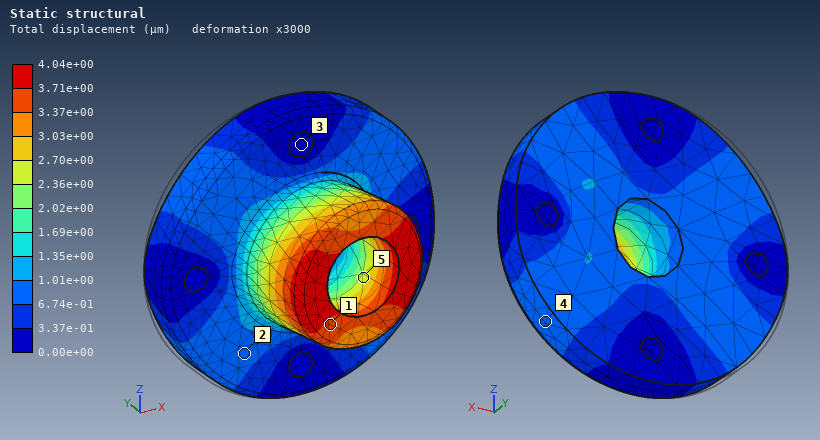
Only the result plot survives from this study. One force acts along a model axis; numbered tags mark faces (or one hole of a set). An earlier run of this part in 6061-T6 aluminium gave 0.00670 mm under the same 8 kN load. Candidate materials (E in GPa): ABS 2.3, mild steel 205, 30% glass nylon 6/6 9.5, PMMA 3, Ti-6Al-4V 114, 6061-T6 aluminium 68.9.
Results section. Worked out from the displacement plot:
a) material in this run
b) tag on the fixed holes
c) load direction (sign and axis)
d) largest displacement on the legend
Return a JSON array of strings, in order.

["Ti-6Al-4V", "3", "+X", "4.04e+00 µm"]
